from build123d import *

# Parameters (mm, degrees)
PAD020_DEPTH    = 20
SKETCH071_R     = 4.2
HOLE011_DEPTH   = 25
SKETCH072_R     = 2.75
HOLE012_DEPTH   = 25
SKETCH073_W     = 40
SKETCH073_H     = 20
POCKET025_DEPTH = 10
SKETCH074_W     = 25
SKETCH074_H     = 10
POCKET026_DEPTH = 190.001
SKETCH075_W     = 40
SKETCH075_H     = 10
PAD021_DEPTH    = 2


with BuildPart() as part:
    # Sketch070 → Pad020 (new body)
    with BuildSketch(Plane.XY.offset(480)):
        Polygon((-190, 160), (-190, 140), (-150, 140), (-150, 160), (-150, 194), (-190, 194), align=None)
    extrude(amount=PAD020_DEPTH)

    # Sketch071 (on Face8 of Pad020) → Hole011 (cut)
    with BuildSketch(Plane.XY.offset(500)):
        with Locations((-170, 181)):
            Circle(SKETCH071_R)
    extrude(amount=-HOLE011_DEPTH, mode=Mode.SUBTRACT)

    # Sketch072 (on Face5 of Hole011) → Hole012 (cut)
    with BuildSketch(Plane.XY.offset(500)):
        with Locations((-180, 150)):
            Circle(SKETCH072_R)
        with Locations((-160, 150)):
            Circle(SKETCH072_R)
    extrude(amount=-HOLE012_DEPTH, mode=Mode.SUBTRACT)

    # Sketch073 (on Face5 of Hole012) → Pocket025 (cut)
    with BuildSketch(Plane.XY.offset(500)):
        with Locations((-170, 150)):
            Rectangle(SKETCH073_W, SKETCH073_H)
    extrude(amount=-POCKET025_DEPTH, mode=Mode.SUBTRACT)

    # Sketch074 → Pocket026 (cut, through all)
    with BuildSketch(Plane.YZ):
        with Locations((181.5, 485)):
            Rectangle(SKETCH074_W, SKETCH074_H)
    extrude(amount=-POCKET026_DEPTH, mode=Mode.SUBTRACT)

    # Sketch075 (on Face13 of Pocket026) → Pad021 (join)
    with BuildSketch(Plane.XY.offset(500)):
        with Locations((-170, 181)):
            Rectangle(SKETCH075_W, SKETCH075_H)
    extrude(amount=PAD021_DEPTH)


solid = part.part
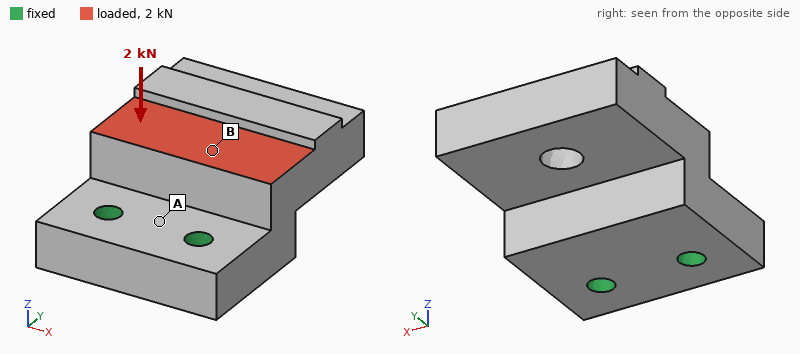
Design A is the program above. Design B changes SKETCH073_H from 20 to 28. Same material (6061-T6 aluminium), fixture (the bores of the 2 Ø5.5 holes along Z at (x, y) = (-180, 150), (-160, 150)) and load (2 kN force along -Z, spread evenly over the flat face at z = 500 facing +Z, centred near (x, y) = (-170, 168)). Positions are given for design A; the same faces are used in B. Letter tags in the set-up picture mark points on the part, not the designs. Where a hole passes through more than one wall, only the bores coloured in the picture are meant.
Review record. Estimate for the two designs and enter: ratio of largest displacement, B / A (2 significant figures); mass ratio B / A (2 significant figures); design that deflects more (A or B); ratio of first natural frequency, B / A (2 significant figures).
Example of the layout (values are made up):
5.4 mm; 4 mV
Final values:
1.5; 0.94; B; 0.83
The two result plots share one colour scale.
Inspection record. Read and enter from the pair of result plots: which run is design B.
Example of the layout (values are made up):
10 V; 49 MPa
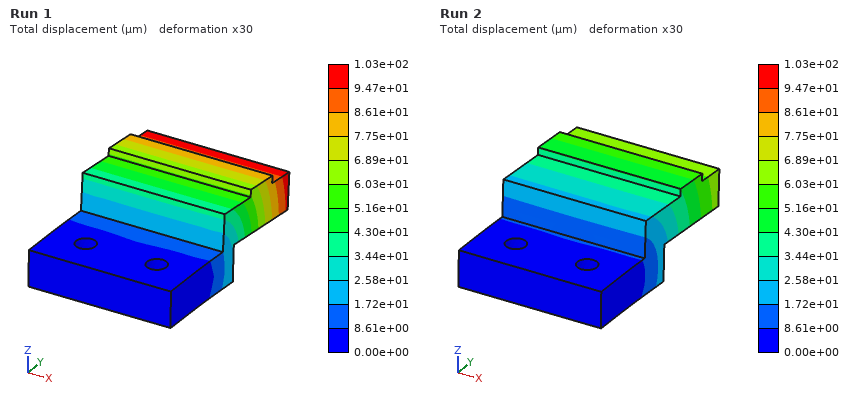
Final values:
Run 1
